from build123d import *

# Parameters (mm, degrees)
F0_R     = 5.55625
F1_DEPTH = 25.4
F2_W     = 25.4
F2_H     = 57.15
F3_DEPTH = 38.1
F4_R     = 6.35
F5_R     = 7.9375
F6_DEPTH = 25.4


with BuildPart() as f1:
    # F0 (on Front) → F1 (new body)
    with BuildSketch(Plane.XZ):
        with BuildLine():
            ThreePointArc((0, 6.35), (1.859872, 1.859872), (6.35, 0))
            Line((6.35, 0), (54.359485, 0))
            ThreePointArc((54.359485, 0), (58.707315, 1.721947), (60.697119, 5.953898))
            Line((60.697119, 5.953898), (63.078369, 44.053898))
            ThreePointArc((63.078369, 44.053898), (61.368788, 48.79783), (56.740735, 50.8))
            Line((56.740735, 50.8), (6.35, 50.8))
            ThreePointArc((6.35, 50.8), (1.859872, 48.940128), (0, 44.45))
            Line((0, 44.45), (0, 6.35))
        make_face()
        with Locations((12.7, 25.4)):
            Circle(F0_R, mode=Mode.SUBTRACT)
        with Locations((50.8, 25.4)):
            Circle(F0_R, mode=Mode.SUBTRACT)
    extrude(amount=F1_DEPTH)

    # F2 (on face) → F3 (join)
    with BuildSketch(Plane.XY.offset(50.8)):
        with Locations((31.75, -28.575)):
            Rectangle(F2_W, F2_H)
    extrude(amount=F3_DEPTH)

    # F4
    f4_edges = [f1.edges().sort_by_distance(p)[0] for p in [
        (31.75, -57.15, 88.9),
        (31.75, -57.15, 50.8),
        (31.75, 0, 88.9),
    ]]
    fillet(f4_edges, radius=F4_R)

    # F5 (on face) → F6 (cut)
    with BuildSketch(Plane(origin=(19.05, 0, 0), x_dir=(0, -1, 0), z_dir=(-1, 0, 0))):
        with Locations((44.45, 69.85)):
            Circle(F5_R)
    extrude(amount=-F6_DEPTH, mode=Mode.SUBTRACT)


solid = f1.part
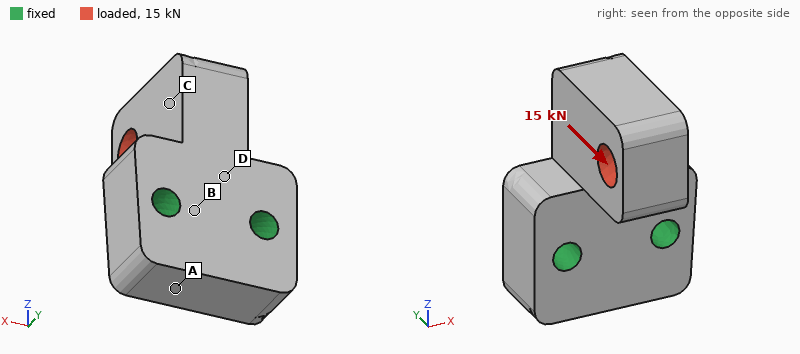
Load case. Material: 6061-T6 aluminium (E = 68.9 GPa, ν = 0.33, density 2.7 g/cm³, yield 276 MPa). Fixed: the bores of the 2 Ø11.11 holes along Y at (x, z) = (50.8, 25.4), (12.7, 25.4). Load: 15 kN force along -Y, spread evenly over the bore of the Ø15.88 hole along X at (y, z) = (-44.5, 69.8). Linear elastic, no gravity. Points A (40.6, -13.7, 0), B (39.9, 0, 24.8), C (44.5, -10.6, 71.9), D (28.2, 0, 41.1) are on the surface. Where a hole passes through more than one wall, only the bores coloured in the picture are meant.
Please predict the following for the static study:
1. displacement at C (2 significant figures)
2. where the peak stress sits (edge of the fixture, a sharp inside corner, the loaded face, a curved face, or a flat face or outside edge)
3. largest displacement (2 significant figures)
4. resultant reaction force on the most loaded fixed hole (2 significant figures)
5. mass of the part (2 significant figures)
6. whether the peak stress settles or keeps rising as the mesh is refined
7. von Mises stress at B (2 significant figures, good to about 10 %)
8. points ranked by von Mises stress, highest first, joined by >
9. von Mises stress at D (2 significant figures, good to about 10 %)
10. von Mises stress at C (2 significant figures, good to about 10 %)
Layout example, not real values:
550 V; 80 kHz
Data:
0.15 mm; edge of the fixture; 0.29 mm; 7.5 kN; 330 g; keeps rising; 49 MPa; D > B > C > A; 97 MPa; 27 MPa
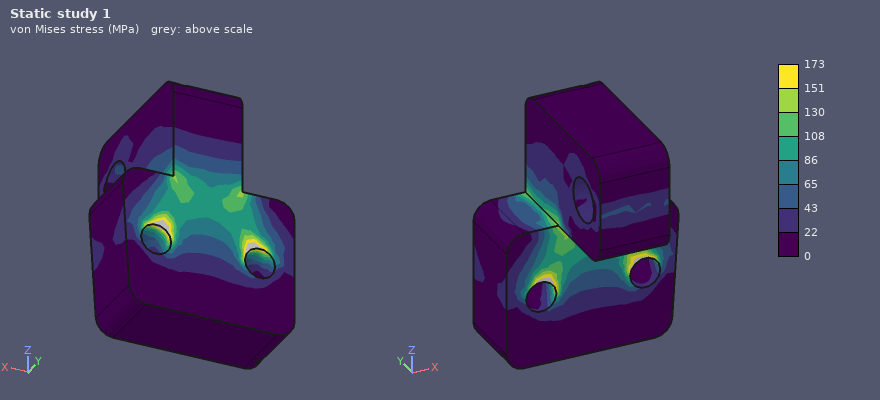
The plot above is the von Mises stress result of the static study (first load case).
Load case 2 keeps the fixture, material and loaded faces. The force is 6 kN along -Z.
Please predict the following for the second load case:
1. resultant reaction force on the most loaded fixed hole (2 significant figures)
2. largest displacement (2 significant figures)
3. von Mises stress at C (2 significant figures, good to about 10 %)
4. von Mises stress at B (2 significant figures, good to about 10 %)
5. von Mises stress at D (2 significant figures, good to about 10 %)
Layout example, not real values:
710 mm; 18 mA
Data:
3.2 kN; 0.15 mm; 16 MPa; 12 MPa; 39 MPa
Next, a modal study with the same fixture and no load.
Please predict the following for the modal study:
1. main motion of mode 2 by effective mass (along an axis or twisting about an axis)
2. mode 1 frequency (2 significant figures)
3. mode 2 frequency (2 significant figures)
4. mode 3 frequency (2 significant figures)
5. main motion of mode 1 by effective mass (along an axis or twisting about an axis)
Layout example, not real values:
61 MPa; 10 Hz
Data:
along X; 3500 Hz; 4900 Hz; 8000 Hz; along Y
